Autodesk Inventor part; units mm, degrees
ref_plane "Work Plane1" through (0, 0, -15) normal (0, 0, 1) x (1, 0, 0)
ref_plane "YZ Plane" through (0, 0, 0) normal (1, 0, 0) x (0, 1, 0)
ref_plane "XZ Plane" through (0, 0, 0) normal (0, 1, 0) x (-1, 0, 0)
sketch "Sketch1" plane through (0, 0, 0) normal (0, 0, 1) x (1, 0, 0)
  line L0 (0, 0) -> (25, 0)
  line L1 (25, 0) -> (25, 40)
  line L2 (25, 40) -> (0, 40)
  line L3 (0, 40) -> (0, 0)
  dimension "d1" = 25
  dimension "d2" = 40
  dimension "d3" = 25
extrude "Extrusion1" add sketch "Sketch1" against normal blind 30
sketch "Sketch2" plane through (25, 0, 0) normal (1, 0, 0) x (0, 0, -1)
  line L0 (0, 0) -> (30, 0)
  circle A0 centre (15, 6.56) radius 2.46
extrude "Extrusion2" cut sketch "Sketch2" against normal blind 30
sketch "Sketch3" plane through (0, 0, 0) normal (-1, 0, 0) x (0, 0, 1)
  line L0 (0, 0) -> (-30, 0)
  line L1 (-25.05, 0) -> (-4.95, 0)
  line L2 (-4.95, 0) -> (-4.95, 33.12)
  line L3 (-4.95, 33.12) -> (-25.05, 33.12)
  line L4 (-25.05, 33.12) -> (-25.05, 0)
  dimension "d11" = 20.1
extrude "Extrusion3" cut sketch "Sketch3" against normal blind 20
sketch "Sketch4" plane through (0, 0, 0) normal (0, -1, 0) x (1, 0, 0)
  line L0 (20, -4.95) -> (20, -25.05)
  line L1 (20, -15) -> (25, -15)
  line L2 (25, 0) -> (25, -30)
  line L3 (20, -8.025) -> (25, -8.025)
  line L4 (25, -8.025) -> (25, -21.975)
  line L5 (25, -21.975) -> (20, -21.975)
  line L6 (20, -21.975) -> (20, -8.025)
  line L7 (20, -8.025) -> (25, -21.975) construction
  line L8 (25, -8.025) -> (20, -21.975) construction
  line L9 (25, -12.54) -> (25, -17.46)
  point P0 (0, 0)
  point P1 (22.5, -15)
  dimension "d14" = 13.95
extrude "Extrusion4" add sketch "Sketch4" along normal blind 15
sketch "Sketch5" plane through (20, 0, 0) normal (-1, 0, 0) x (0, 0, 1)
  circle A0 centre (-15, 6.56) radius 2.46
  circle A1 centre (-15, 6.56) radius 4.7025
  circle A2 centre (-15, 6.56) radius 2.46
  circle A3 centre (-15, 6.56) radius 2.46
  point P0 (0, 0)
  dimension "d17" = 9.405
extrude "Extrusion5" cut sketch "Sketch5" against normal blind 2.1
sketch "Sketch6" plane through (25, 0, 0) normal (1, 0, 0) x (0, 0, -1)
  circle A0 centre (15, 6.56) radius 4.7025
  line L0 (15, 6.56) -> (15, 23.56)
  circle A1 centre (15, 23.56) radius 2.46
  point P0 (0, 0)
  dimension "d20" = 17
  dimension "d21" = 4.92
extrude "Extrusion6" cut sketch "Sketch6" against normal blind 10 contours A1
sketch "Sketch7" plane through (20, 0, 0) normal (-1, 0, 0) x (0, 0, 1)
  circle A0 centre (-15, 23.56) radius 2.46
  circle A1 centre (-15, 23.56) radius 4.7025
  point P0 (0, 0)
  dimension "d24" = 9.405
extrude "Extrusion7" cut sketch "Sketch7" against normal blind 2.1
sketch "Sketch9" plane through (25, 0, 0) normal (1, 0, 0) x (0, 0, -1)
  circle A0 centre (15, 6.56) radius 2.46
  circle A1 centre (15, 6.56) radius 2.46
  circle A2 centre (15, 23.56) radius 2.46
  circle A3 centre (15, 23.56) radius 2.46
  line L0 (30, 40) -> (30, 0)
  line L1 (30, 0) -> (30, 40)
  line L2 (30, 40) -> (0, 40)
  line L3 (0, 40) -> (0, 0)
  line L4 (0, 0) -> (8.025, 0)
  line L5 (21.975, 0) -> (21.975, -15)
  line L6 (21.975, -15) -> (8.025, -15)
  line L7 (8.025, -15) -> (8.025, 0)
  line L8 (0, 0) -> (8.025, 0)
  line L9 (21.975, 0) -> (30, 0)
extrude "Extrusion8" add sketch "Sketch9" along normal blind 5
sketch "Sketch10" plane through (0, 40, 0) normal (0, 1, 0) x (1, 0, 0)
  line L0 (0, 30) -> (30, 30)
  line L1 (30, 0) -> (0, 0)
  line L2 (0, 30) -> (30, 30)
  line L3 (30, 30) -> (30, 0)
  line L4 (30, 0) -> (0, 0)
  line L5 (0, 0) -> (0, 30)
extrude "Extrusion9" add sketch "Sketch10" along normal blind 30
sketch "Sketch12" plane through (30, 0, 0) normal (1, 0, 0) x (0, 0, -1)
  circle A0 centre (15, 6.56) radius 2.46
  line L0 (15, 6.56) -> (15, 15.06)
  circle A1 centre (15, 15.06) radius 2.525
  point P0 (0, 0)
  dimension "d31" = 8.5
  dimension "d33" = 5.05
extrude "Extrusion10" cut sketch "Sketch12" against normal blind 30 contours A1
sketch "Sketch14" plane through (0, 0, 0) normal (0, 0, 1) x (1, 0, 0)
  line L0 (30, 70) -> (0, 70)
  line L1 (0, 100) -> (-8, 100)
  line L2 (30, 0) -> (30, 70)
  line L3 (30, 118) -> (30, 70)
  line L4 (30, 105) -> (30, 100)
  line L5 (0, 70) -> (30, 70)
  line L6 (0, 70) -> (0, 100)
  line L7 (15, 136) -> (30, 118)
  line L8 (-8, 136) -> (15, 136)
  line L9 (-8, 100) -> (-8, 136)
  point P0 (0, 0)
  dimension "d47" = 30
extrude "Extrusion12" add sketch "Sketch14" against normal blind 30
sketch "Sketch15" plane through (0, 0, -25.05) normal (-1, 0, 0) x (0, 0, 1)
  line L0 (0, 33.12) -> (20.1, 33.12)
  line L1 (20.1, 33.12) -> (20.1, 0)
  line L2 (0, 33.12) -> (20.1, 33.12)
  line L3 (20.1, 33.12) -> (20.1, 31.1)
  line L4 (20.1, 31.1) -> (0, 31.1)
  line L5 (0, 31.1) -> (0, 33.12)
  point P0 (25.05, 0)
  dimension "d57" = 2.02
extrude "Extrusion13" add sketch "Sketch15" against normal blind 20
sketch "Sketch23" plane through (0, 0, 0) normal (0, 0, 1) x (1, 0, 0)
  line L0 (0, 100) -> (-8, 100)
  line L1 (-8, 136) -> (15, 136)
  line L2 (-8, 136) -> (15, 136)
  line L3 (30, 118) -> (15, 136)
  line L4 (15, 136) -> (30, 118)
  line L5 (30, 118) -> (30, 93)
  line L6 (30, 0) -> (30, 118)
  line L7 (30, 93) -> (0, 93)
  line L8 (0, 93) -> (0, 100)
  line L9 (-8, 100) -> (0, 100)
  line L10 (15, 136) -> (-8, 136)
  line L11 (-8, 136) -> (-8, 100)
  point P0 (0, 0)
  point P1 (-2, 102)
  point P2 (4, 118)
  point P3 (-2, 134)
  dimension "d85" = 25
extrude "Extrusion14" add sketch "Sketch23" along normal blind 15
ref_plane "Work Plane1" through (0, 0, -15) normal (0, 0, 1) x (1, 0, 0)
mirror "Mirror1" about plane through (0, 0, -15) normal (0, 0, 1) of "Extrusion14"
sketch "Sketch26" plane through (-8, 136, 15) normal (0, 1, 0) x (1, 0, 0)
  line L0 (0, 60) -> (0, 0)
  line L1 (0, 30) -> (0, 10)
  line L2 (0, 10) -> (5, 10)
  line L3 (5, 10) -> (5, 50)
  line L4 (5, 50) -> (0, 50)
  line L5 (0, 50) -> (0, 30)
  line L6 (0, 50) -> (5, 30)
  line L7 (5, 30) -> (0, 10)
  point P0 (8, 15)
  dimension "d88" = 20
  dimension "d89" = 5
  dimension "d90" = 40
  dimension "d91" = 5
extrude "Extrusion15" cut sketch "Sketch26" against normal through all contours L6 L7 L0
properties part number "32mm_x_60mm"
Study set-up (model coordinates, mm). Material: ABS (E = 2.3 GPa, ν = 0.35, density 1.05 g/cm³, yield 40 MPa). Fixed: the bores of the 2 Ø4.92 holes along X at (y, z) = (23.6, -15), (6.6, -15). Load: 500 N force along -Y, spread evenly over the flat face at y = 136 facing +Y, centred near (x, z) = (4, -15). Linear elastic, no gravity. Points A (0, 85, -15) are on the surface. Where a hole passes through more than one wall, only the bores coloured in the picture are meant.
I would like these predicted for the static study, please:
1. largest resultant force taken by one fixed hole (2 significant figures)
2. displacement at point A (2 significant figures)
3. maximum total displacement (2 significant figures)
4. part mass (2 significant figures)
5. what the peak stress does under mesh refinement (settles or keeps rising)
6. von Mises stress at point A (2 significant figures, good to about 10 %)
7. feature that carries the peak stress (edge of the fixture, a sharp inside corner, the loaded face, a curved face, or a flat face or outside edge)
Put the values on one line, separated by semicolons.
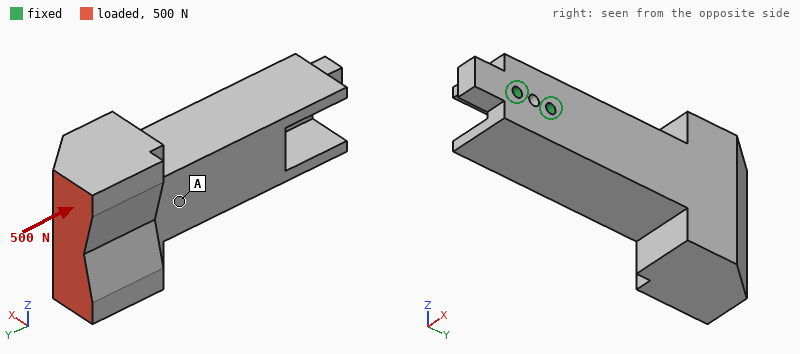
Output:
500 N; 0.53 mm; 1.0 mm; 160 g; keeps rising; 1.6 MPa; edge of the fixture
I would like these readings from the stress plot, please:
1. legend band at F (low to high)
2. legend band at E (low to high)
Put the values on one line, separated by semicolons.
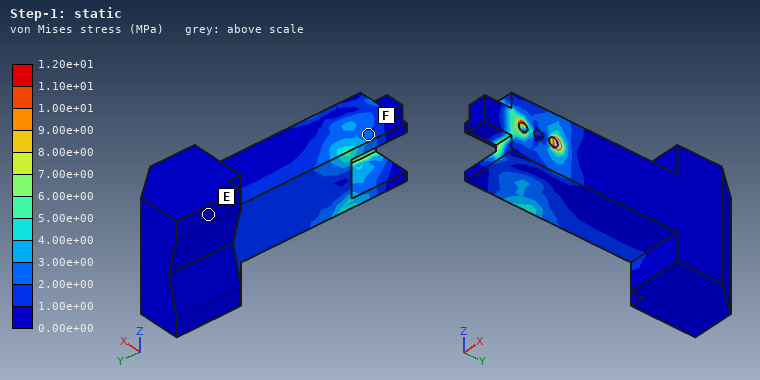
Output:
2.00e+00 to 3.00e+00 MPa; 0.00e+00 to 1.00e+00 MPa
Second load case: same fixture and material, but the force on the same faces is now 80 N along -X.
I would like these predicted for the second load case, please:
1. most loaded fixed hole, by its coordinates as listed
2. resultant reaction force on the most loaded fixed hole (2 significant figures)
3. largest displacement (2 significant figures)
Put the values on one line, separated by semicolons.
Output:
(23.6, -15); 440 N; 0.92 mm
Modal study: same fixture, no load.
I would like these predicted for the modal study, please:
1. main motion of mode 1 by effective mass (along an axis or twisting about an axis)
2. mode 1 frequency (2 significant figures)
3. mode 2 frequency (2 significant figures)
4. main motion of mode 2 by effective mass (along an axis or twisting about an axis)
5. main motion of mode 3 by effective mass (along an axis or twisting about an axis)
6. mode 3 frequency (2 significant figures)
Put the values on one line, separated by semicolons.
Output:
along X; 190 Hz; 220 Hz; along Z; twisting about Y; 530 Hz
